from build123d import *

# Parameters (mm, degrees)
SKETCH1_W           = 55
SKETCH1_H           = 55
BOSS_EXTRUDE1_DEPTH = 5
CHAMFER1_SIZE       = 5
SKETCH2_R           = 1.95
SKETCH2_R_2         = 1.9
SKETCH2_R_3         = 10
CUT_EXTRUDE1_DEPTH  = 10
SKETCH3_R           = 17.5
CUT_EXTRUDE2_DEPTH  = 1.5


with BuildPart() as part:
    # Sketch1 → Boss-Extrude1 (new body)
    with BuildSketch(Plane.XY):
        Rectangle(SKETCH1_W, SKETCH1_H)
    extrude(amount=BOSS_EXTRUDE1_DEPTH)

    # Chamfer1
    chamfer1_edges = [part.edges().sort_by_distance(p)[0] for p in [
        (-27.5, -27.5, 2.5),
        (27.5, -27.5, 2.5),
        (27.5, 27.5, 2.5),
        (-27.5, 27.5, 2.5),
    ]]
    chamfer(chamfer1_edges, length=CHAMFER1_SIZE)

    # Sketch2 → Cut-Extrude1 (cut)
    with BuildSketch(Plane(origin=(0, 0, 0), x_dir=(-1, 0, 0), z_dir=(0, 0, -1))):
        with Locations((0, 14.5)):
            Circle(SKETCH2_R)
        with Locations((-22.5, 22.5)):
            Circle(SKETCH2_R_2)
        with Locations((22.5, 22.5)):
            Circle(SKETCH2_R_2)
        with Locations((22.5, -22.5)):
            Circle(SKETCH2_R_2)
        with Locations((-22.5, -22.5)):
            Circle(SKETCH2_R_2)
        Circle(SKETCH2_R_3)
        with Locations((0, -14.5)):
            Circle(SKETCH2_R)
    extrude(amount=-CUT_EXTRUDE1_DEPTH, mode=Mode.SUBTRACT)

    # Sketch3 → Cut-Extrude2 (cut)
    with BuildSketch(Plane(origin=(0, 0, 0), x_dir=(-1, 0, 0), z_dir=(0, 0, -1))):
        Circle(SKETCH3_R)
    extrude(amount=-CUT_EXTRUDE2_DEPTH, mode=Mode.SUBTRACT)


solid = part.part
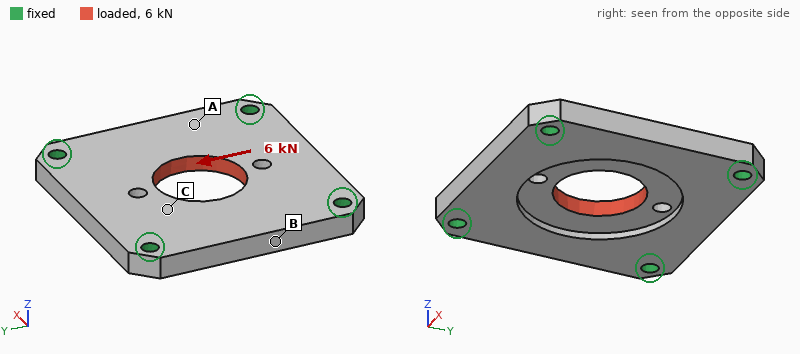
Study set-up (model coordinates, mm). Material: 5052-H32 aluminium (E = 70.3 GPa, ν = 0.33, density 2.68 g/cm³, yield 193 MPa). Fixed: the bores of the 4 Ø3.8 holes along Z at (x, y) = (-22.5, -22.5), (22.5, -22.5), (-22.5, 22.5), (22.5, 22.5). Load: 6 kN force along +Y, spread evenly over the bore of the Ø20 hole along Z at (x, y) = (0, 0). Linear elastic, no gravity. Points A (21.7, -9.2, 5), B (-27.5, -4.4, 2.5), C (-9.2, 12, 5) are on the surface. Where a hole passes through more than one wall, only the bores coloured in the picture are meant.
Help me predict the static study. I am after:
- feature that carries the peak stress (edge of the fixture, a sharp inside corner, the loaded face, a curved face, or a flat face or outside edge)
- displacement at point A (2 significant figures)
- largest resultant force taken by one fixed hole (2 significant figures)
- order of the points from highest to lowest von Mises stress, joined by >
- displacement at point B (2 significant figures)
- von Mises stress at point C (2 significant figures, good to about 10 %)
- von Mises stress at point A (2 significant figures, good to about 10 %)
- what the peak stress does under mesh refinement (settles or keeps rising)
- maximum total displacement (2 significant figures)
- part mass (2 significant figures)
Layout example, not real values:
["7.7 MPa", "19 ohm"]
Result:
["edge of the fixture", "3.6 µm", "1.6 kN", "C > A > B", "3.4 µm", "25 MPa", "14 MPa", "keeps rising", "17 µm", "32 g"]
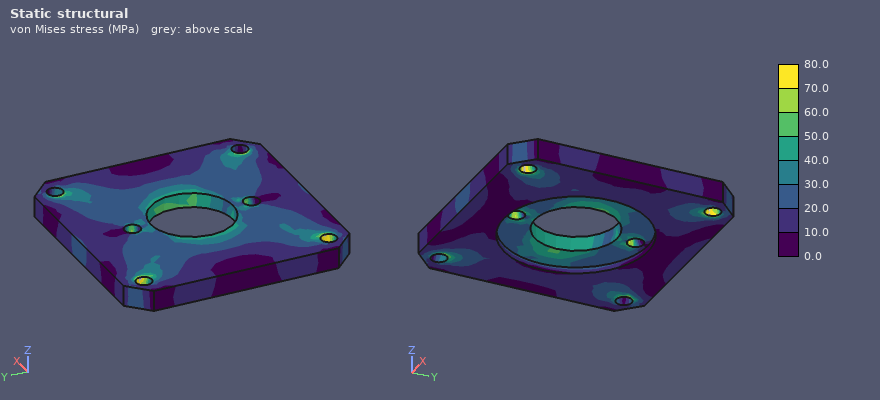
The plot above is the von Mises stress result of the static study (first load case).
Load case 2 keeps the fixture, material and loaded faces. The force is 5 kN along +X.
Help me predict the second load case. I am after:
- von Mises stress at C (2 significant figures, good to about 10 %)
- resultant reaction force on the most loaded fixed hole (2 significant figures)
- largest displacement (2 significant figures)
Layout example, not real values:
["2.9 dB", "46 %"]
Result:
["22 MPa", "1.4 kN", "14 µm"]
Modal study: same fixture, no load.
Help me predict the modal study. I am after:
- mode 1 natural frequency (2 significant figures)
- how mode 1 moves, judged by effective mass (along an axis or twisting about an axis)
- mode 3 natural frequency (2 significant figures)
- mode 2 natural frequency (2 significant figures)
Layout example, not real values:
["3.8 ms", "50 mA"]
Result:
["9200 Hz", "along Z", "13 kHz", "13 kHz"]
